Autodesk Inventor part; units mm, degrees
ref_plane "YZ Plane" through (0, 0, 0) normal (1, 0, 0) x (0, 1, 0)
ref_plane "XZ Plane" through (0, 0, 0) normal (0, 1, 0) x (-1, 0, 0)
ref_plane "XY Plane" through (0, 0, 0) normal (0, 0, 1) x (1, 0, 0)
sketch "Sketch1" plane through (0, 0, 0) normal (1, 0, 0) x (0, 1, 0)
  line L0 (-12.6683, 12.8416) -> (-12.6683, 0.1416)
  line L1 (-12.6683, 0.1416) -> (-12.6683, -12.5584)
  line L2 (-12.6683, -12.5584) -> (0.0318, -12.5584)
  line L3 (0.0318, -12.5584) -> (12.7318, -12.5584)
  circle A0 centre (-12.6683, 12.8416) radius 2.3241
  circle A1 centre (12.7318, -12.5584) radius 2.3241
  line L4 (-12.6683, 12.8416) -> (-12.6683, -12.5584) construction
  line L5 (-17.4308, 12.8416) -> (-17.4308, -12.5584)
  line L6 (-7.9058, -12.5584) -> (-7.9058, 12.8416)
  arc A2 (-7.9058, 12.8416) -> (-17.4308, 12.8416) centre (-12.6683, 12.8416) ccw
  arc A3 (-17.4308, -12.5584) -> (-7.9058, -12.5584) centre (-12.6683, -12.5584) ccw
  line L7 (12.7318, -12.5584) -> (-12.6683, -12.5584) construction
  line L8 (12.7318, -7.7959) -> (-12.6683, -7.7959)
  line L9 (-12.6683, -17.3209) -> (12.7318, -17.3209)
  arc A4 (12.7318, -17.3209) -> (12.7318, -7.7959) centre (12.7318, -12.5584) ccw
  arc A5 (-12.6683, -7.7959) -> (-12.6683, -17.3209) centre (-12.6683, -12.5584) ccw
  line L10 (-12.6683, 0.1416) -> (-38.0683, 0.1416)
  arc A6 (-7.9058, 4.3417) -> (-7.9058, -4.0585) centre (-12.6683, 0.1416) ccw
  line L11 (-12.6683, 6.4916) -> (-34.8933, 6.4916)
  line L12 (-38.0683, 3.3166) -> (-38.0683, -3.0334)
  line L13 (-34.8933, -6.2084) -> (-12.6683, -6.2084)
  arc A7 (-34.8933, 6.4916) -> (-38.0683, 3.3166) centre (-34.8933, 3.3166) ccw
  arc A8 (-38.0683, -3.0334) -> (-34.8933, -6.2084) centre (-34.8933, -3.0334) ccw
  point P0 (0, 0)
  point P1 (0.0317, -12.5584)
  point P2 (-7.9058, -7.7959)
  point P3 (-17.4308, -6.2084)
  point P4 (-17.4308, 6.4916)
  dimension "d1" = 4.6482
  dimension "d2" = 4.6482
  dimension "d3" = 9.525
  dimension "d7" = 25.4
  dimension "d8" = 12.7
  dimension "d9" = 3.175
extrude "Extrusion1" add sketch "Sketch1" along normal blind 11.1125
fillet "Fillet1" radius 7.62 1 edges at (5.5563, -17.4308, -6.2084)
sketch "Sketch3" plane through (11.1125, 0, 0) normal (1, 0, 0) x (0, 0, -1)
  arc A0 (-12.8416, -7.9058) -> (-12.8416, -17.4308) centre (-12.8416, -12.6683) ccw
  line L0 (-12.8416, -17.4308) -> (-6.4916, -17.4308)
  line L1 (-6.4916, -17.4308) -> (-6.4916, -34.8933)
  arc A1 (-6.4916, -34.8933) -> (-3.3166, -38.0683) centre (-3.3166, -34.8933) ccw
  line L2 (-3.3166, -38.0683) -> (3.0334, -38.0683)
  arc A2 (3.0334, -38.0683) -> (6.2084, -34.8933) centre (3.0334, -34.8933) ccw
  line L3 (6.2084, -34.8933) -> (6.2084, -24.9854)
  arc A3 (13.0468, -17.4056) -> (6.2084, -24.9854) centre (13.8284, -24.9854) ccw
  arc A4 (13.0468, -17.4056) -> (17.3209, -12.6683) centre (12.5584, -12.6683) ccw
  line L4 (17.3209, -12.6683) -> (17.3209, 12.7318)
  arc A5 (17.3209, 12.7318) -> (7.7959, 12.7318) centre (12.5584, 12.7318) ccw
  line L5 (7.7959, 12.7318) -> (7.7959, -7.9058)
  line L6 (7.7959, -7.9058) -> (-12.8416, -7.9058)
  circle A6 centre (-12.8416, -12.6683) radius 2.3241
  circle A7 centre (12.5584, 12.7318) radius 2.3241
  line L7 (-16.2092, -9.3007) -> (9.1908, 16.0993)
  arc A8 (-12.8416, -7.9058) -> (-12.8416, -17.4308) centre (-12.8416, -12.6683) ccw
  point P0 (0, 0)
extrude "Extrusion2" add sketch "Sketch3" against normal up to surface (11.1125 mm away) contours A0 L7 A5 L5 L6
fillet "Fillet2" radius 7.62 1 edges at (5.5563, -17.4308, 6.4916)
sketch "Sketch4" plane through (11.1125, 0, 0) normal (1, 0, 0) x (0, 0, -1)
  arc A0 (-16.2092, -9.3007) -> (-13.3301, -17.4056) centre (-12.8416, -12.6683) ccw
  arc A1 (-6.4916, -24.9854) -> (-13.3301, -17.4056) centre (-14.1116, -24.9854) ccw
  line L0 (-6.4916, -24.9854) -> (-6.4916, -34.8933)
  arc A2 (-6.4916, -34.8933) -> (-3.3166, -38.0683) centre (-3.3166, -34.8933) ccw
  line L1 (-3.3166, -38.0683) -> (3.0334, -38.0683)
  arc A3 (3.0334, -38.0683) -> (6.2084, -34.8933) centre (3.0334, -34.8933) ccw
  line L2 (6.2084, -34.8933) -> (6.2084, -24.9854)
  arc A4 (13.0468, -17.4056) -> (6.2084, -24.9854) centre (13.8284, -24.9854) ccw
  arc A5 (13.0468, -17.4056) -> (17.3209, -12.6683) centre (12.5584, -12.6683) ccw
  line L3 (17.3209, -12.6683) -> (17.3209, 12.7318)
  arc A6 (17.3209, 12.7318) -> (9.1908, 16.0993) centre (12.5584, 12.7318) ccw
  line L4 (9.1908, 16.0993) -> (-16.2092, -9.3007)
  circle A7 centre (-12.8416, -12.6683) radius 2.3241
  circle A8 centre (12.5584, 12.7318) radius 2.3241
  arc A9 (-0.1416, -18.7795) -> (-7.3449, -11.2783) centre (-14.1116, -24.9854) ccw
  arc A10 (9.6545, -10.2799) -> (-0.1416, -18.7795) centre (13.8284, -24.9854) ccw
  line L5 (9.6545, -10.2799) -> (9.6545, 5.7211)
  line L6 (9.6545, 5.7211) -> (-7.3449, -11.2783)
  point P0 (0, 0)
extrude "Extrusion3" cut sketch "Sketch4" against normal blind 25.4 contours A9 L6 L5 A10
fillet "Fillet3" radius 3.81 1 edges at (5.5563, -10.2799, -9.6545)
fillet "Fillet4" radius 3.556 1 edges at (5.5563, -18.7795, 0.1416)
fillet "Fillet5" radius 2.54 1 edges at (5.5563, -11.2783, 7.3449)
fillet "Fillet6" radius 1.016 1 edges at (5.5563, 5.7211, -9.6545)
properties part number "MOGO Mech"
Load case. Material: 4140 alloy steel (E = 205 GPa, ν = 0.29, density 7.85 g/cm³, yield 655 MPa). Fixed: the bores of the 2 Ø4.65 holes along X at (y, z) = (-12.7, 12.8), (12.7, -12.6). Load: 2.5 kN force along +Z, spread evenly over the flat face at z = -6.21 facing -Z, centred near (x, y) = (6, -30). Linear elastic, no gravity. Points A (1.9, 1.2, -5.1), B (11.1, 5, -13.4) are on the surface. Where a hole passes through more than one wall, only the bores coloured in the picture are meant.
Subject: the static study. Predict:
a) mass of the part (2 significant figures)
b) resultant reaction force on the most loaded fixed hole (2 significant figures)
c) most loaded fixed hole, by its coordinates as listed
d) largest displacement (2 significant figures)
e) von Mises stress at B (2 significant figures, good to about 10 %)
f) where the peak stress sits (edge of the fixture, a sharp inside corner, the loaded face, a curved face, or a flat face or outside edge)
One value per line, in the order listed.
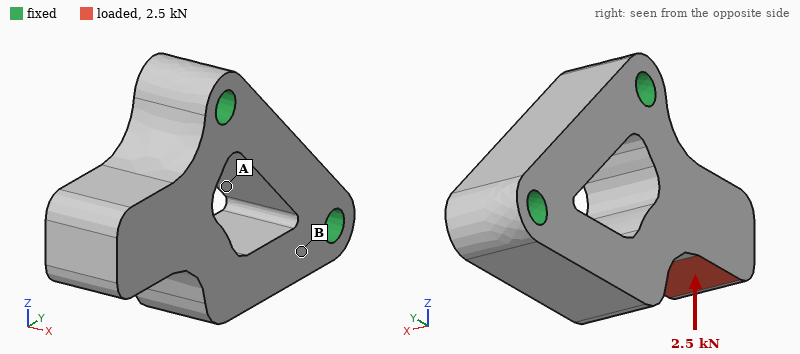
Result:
77 g
2.8 kN
(-12.7, 12.8)
17 µm
25 MPa
a curved face
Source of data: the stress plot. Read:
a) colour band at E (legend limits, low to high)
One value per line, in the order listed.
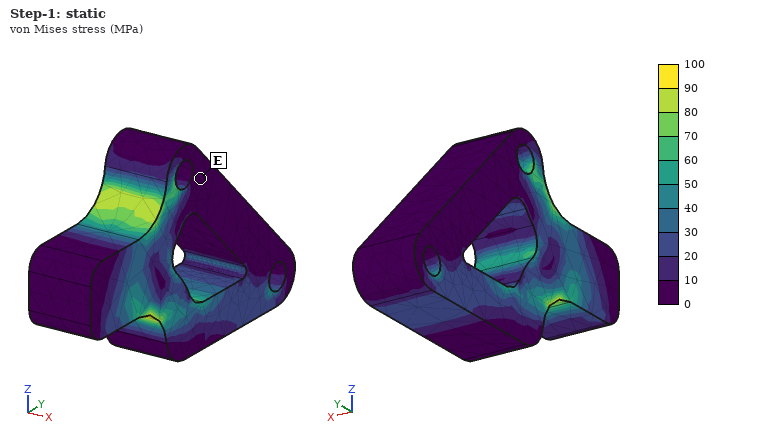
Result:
0 to 10 MPa
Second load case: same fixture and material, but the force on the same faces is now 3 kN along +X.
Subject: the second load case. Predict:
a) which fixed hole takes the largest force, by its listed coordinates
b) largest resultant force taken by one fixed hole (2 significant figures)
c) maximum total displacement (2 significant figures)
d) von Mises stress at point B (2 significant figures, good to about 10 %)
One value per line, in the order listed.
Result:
(-12.7, 12.8)
2.8 kN
86 µm
92 MPa
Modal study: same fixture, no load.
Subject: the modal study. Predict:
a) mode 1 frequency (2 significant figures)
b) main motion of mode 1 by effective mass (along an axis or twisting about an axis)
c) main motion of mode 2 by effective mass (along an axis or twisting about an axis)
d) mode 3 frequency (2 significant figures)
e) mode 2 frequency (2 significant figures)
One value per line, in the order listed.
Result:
8600 Hz
along X
along Z
16 kHz
15 kHz
